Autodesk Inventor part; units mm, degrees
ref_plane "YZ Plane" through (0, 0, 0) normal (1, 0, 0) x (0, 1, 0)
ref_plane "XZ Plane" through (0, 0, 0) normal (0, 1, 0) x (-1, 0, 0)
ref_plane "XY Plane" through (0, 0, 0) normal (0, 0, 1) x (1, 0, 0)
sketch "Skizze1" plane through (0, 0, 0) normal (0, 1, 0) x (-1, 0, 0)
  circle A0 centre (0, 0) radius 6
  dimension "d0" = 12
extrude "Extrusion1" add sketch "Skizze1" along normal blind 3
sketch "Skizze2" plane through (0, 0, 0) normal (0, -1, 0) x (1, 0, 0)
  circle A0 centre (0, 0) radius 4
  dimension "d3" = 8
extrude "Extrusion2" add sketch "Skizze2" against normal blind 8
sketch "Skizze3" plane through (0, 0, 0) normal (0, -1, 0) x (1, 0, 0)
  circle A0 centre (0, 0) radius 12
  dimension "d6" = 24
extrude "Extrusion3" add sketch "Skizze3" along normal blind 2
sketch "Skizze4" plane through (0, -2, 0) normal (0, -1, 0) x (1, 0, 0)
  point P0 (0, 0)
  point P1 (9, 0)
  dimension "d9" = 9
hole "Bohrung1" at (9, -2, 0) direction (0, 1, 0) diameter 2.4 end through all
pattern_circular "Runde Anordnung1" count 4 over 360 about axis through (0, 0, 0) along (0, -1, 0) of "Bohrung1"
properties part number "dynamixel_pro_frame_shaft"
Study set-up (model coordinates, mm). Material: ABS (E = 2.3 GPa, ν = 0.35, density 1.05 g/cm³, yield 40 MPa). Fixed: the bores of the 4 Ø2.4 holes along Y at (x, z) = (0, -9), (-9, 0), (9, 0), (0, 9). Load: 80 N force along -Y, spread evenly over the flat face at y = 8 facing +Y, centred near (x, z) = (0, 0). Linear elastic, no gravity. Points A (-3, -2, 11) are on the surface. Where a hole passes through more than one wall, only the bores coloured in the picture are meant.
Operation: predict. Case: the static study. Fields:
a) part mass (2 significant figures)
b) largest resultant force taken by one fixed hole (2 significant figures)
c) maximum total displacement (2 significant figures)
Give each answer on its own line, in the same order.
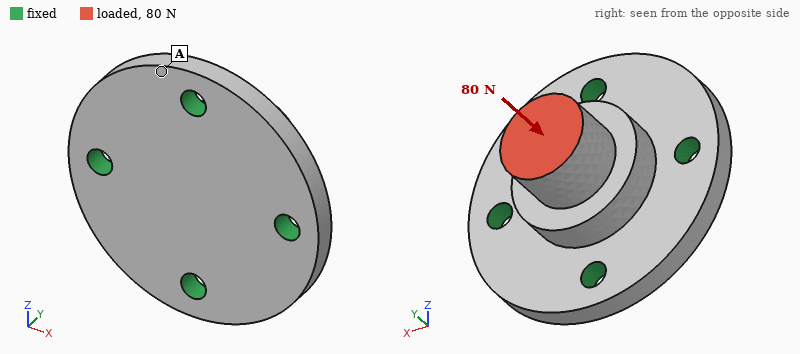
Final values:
1.5 g
22 N
19 µm
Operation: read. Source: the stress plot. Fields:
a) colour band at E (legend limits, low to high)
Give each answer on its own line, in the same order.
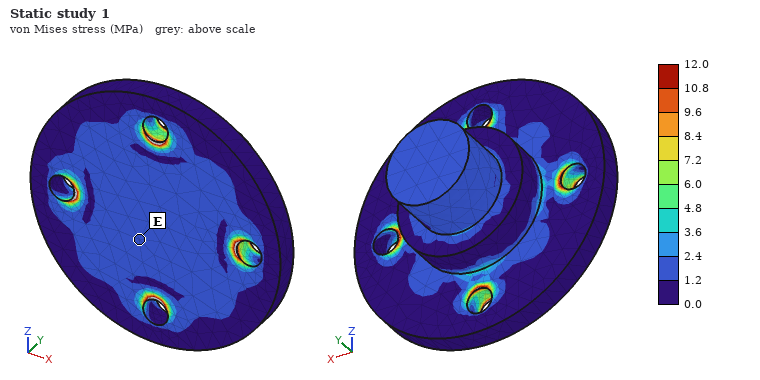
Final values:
1.2 to 2.4 MPa
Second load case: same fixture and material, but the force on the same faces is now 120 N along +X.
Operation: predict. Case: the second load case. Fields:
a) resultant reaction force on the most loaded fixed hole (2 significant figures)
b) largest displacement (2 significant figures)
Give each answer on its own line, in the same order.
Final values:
82 N
0.11 mm
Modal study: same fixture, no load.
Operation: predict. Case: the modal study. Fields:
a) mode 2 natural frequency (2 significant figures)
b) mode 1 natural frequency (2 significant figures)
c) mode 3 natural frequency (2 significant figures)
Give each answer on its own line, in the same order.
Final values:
12 kHz
12 kHz
12 kHz
